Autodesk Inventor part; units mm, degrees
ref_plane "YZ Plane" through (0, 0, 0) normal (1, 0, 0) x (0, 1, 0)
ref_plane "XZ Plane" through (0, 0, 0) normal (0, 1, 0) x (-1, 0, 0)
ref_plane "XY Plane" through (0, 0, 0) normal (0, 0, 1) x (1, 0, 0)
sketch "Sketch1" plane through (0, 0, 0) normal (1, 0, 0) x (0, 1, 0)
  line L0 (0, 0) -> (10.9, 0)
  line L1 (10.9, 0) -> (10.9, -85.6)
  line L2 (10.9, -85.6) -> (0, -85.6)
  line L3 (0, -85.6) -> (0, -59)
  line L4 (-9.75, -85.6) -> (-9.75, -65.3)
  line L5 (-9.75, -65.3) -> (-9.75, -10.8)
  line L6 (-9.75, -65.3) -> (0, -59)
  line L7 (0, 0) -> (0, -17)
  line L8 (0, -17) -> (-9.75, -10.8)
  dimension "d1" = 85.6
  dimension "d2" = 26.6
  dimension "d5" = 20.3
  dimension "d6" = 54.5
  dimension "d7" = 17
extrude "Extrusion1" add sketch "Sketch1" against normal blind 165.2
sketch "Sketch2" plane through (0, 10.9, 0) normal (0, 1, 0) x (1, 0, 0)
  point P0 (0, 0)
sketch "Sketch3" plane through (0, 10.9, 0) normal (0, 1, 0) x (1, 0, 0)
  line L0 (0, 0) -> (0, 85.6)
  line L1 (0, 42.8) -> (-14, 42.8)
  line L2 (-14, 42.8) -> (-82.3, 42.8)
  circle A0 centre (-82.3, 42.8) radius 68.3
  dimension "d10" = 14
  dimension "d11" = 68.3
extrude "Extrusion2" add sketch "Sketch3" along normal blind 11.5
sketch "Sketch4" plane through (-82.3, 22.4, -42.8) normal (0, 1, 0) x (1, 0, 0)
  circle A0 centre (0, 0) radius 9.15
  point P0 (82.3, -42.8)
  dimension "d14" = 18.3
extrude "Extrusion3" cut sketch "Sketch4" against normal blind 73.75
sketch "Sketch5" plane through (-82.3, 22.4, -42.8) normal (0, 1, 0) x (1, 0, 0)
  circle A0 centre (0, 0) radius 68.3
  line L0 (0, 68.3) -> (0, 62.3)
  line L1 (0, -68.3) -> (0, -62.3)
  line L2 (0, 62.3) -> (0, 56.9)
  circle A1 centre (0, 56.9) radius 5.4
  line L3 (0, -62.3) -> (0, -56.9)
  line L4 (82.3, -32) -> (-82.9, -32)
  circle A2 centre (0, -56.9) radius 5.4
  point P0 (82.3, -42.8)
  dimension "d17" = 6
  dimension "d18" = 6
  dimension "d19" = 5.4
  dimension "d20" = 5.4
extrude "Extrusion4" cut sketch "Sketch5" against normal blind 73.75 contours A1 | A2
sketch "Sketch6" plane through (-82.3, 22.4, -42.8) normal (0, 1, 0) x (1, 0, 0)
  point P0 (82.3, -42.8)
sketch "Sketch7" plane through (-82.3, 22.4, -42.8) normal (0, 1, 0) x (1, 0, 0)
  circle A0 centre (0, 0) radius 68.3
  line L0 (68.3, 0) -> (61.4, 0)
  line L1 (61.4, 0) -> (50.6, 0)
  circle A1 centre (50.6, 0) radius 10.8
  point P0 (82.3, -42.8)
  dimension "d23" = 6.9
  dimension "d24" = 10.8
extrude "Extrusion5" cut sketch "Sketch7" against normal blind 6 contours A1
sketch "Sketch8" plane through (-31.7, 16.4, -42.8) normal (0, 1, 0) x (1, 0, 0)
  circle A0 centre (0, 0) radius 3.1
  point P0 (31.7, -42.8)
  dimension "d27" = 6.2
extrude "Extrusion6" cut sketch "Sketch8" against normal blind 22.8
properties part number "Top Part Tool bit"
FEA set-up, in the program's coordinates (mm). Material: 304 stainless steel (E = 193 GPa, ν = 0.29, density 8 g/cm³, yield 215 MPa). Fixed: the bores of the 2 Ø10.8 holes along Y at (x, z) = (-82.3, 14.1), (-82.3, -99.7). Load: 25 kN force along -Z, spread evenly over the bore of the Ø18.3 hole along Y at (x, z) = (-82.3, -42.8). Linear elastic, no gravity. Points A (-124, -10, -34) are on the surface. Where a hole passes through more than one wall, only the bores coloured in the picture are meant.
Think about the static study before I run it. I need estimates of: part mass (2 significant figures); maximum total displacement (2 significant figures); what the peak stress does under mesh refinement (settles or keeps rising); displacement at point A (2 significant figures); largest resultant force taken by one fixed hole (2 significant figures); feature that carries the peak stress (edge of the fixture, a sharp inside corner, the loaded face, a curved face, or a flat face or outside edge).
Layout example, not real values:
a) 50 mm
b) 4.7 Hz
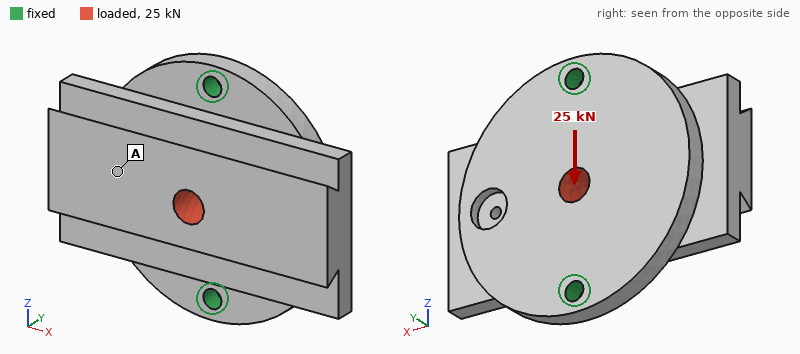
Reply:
a) 3.1 kg
b) 8.2 µm
c) keeps rising
d) 5.0 µm
e) 13 kN
f) edge of the fixture
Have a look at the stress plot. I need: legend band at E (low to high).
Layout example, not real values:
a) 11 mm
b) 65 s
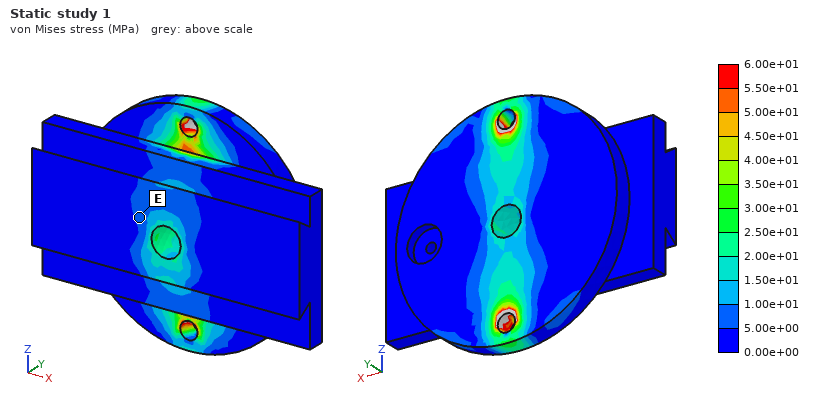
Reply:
a) 5.00e+00 to 1.00e+01 MPa
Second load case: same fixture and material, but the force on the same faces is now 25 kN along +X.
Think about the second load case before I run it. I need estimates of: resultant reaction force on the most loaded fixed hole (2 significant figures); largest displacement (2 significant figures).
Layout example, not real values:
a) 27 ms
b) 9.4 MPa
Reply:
a) 13 kN
b) 98 µm
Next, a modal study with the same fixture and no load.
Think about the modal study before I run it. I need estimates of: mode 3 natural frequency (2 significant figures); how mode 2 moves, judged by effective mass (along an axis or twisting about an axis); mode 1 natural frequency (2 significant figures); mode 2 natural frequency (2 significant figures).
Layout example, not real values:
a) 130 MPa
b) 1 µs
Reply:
a) 5400 Hz
b) along Y
c) 1000 Hz
d) 2600 Hz
